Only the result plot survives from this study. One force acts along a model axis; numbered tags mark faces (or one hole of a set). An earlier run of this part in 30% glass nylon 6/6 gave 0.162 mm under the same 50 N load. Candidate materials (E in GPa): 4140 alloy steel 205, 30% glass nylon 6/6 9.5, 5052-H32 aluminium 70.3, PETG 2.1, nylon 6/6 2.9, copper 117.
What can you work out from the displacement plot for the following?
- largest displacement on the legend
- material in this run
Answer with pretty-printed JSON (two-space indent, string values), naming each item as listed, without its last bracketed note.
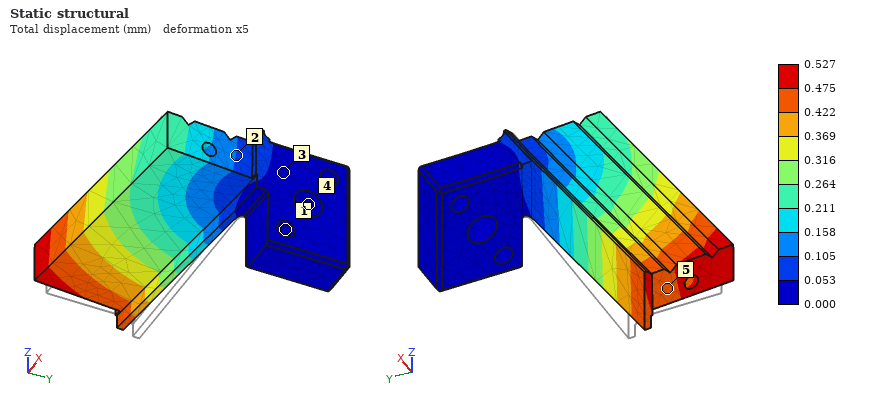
{
  "largest displacement on the legend": "0.527 mm",
  "material in this run": "nylon 6/6"
}
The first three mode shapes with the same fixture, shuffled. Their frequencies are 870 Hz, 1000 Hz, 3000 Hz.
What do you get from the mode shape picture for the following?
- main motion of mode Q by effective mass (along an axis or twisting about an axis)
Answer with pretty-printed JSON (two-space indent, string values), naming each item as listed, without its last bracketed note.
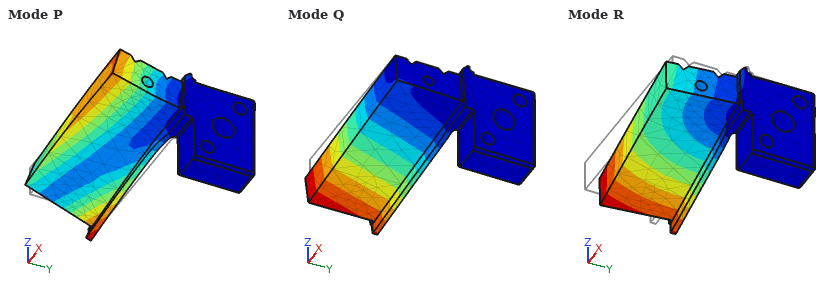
{
  "main motion of mode Q by effective mass": "along Z"
}
